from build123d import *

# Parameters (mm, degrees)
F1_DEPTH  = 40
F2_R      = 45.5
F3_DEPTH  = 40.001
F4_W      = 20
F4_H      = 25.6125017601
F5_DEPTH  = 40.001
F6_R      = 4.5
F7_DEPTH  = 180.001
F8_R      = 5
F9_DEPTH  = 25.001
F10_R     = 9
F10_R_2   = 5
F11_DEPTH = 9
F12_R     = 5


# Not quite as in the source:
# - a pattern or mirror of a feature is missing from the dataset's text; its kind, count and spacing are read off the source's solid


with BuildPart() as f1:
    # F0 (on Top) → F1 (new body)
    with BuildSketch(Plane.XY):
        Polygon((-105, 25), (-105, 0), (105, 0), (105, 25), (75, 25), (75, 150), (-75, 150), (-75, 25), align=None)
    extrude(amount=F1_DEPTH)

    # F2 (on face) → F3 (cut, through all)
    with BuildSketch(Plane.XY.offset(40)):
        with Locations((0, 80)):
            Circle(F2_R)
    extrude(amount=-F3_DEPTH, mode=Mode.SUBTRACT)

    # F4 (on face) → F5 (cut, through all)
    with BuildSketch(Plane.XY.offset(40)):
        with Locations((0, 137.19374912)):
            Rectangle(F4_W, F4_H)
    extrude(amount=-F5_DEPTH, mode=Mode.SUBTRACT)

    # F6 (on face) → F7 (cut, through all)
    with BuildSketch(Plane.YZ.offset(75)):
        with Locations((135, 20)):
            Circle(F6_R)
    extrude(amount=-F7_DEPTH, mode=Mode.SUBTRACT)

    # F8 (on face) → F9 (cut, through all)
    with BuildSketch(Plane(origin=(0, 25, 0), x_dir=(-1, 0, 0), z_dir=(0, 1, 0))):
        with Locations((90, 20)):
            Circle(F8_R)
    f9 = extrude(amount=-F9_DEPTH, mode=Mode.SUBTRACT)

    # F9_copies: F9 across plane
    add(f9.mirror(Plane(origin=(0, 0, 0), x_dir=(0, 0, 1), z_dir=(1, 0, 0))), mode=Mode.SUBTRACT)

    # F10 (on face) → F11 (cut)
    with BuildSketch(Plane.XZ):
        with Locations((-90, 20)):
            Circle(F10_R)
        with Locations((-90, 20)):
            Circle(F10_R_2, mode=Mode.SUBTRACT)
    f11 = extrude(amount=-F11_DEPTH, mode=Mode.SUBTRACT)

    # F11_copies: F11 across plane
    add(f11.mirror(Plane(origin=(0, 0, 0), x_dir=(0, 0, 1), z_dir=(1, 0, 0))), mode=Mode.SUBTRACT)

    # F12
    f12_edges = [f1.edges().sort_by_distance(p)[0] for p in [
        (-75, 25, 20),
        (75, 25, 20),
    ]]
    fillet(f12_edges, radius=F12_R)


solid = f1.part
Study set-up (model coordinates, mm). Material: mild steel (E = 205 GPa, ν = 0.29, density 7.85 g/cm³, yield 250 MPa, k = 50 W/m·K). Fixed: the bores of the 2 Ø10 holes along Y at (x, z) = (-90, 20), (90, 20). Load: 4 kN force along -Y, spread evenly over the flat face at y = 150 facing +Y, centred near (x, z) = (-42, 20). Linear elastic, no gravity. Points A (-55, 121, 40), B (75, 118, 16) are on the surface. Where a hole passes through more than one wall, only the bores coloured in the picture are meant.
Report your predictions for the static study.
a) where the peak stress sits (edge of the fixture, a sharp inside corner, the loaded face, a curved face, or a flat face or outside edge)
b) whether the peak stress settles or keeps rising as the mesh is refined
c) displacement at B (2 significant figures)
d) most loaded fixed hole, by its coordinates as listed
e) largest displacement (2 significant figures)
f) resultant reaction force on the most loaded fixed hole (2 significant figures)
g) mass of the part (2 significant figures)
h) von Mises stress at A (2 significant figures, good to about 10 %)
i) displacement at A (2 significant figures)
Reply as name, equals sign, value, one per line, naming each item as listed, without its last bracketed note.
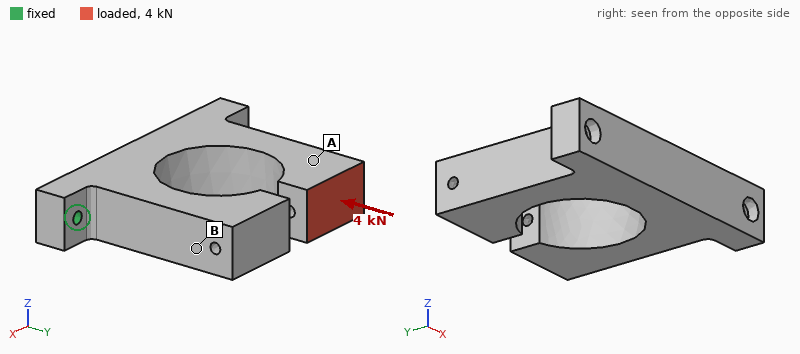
where the peak stress sits = edge of the fixture
whether the peak stress settles or keeps rising as the mesh is refined = keeps rising
displacement at B = 7.1 µm
most loaded fixed hole, by its coordinates as listed = (-90, 20)
largest displacement = 32 µm
resultant reaction force on the most loaded fixed hole = 3.1 kN
mass of the part = 5.2 kg
von Mises stress at A = 3.6 MPa
displacement at A = 17 µm
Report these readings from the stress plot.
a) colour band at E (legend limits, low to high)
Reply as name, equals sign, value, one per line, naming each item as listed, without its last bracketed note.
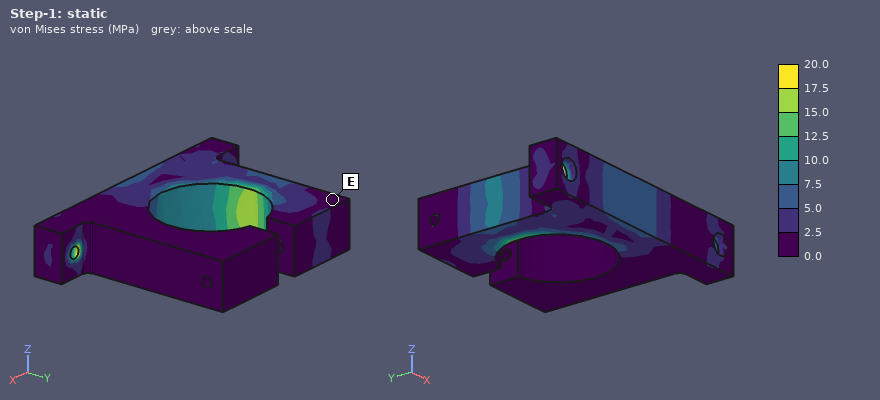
colour band at E = 0.0 to 2.5 MPa
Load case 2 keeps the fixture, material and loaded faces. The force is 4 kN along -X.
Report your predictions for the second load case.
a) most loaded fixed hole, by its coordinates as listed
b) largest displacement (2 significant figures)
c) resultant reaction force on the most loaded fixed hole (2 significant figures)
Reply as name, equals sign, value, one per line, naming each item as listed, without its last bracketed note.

most loaded fixed hole, by its coordinates as listed = (90, 20)
largest displacement = 0.14 mm
resultant reaction force on the most loaded fixed hole = 4.7 kN
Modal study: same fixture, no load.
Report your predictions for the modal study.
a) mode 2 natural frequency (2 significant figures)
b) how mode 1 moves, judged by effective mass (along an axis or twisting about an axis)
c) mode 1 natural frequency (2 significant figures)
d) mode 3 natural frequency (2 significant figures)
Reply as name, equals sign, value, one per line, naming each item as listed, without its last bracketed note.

mode 2 natural frequency = 1000 Hz
how mode 1 moves, judged by effective mass = along Z
mode 1 natural frequency = 650 Hz
mode 3 natural frequency = 1000 Hz
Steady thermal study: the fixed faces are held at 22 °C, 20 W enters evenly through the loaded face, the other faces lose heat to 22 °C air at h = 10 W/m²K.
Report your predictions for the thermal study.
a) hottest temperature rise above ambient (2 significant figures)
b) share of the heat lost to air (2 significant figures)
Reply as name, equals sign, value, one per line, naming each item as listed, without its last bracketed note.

hottest temperature rise above ambient = 35 K
share of the heat lost to air = 33 %
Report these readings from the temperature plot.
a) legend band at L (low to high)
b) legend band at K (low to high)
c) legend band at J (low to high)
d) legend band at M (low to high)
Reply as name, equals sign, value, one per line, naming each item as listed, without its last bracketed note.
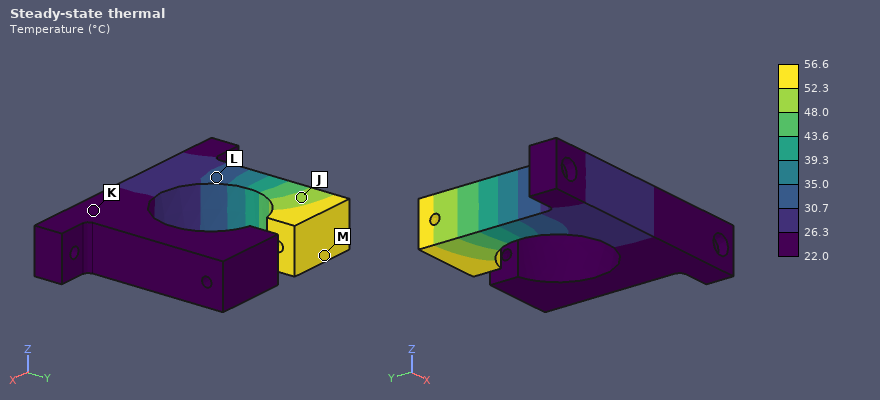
legend band at L = 30.7 to 35.0 °C
legend band at K = 22.0 to 26.3 °C
legend band at J = 48.0 to 52.3 °C
legend band at M = 52.3 to 56.6 °C
